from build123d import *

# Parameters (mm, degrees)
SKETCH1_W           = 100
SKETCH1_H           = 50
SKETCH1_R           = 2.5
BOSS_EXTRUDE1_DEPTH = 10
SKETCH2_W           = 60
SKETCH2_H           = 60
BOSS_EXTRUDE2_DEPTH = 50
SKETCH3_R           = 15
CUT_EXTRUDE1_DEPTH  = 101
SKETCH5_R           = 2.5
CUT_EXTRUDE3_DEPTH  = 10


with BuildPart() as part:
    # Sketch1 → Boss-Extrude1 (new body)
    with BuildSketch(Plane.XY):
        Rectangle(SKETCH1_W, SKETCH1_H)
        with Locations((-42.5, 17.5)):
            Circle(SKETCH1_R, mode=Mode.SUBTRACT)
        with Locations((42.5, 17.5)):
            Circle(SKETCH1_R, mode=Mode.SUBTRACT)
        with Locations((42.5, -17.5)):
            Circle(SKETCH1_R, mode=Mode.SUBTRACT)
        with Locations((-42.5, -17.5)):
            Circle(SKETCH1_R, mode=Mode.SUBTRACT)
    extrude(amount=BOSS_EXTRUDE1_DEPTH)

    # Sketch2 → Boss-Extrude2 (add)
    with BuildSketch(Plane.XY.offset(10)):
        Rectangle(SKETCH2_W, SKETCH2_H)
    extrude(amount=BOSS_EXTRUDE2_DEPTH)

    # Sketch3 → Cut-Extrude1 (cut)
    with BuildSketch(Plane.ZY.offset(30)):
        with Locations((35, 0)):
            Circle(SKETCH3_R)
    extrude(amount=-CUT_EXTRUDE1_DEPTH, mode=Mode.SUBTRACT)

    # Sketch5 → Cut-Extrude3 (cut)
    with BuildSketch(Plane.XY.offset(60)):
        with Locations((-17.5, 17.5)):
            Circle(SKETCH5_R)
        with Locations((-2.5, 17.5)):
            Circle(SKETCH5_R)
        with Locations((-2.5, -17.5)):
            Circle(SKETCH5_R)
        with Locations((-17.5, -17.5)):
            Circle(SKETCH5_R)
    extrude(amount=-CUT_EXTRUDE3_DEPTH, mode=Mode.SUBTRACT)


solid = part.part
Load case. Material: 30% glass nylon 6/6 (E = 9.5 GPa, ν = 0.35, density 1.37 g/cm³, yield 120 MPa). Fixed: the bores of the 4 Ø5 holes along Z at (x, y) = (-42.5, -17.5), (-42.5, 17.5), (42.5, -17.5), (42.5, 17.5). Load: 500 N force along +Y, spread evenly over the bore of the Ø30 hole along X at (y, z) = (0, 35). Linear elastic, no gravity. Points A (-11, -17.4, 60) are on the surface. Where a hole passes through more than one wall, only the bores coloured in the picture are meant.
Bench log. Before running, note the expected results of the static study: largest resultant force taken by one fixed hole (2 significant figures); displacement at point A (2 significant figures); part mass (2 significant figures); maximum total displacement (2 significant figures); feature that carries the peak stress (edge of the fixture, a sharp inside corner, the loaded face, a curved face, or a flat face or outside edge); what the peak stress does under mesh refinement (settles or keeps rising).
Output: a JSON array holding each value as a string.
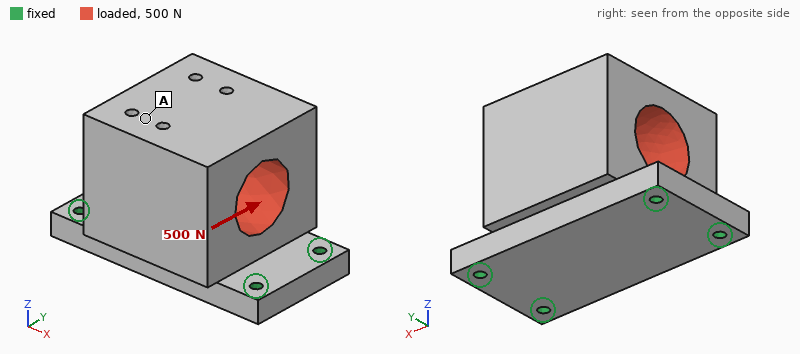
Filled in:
["280 N", "47 µm", "250 g", "50 µm", "edge of the fixture", "keeps rising"]
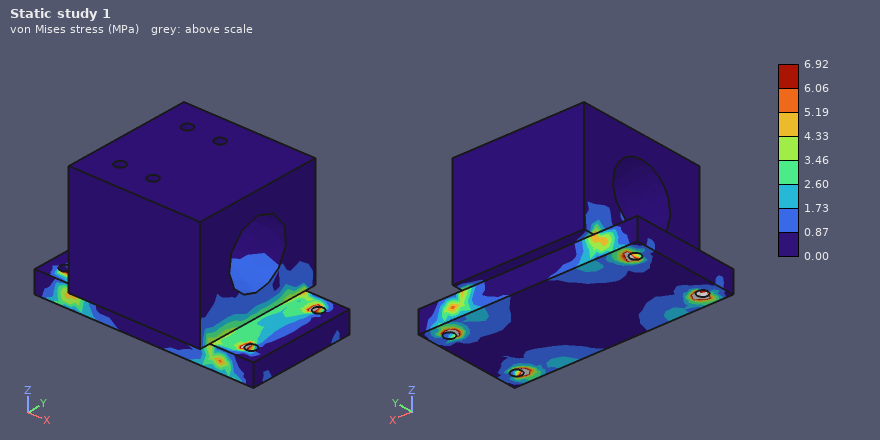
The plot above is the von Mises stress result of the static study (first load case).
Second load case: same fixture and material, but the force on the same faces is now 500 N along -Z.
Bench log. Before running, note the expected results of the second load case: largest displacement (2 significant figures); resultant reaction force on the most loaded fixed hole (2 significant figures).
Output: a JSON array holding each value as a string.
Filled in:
["9.1 µm", "140 N"]
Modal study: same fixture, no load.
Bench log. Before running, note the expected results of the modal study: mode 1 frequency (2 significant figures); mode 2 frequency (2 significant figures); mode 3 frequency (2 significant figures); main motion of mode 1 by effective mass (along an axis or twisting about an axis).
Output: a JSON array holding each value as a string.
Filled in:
["1300 Hz", "2600 Hz", "2700 Hz", "along Y"]
